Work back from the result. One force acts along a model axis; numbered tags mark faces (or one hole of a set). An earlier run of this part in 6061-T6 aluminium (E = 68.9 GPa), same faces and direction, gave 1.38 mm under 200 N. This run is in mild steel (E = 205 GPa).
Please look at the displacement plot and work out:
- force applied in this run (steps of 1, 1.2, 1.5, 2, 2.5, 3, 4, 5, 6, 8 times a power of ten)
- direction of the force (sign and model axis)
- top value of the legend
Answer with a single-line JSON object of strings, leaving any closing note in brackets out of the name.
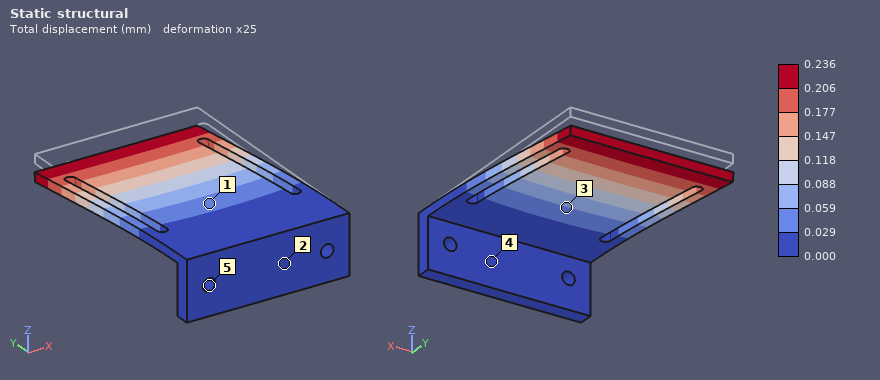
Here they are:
{"force applied in this run": "100 N", "direction of the force": "-Z", "top value of the legend": "0.236 mm"}
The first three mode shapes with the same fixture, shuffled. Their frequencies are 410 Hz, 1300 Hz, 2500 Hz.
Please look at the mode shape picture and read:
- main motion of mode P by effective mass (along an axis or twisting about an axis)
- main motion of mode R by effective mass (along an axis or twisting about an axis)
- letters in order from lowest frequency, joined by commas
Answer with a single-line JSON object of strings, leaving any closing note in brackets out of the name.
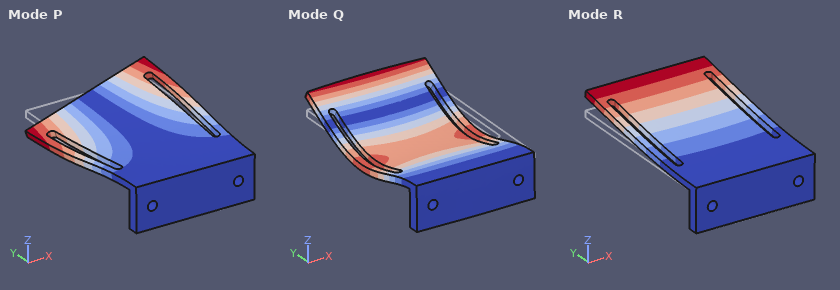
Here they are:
{"main motion of mode P by effective mass": "twisting about Y", "main motion of mode R by effective mass": "along Z", "letters in order from lowest frequency, joined by commas": "R, P, Q"}
